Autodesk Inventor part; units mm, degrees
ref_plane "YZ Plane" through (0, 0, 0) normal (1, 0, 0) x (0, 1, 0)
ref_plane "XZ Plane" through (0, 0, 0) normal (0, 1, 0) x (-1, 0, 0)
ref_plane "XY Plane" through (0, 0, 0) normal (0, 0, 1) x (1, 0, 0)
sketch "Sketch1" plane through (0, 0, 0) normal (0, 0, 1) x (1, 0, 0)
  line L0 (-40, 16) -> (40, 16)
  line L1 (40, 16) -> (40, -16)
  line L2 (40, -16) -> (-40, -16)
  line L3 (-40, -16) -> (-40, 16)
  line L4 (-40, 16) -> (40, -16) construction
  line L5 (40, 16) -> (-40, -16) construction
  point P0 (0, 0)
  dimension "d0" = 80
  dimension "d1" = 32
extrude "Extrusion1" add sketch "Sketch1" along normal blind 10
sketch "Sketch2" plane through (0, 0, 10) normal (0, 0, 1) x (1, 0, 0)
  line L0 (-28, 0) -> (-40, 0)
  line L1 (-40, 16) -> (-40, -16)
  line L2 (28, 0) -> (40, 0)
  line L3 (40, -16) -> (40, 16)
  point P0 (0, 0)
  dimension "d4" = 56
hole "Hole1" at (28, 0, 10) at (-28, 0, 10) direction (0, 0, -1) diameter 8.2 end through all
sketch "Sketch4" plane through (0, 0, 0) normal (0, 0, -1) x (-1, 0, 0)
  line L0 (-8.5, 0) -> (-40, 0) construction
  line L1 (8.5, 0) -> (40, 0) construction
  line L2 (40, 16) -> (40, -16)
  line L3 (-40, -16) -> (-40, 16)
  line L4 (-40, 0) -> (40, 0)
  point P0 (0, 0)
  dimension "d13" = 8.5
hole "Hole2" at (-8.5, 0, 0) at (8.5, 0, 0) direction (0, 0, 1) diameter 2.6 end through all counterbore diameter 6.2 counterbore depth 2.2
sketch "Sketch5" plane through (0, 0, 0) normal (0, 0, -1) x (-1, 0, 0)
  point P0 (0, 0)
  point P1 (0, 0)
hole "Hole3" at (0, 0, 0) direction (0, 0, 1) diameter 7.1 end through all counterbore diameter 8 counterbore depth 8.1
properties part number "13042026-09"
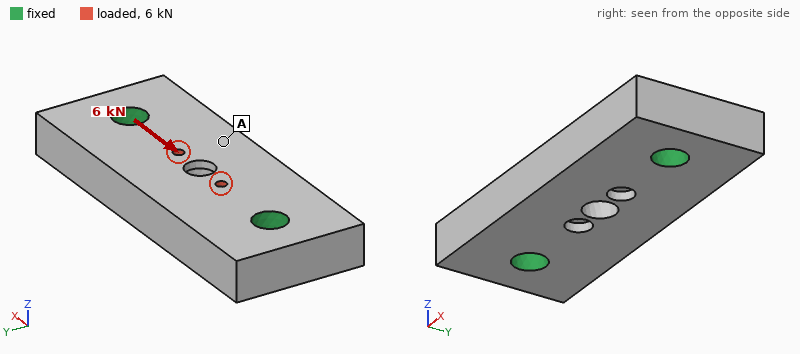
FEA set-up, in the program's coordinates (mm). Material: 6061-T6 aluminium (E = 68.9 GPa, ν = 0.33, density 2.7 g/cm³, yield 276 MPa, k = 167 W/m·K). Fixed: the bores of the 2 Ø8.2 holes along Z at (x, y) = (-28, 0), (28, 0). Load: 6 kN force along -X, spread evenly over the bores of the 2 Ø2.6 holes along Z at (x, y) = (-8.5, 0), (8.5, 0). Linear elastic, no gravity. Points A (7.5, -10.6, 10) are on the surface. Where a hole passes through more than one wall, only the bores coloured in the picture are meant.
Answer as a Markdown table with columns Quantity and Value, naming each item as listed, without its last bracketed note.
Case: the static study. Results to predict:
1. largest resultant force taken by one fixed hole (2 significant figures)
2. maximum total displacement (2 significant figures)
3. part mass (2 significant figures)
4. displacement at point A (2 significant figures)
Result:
| Quantity | Value |
|---|---|
| largest resultant force taken by one fixed hole | 3.0 kN |
| maximum total displacement | 7.2 µm |
| part mass | 64 g |
| displacement at point A | 2.8 µm |
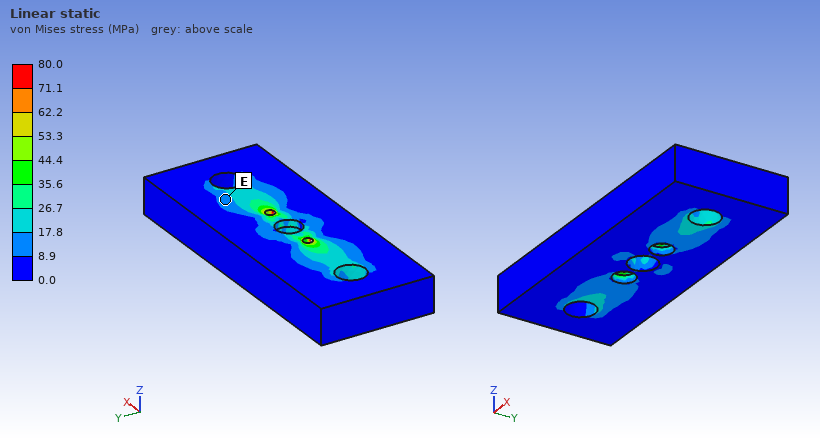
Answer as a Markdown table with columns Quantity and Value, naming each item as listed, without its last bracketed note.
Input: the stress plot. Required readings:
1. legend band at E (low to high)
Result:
| Quantity | Value |
|---|---|
| legend band at E | 8.9 to 17.8 MPa |
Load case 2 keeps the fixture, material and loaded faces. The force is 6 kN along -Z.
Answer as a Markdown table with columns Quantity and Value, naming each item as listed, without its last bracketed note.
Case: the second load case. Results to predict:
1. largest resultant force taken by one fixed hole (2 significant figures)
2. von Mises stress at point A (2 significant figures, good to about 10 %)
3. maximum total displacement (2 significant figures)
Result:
| Quantity | Value |
|---|---|
| largest resultant force taken by one fixed hole | 3.0 kN |
| von Mises stress at point A | 34 MPa |
| maximum total displacement | 36 µm |
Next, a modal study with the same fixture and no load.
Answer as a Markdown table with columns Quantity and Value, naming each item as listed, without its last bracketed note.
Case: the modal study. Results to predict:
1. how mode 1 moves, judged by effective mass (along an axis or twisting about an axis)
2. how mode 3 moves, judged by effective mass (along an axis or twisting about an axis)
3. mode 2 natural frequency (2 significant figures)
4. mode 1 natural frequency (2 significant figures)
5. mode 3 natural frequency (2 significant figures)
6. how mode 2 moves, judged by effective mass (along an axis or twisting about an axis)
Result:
| Quantity | Value |
|---|---|
| how mode 1 moves, judged by effective mass | along Z |
| how mode 3 moves, judged by effective mass | along Y |
| mode 2 natural frequency | 16 kHz |
| mode 1 natural frequency | 14 kHz |
| mode 3 natural frequency | 21 kHz |
| how mode 2 moves, judged by effective mass | twisting about X |
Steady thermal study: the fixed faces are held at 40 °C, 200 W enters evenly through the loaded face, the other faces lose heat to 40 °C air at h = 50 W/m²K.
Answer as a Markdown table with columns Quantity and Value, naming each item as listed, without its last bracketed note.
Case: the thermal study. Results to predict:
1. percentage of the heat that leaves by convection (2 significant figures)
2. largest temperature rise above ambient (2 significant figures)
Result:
| Quantity | Value |
|---|---|
| percentage of the heat that leaves by convection | 3.2 % |
| largest temperature rise above ambient | 57 K |
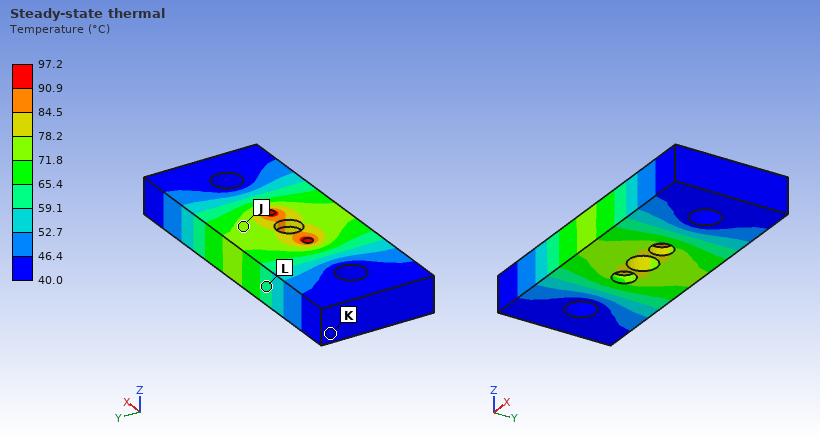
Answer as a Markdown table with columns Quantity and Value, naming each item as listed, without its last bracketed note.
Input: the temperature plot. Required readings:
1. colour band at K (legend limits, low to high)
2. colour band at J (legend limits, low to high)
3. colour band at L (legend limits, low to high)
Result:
| Quantity | Value |
|---|---|
| colour band at K | 40.0 to 46.4 °C |
| colour band at J | 71.8 to 78.2 °C |
| colour band at L | 59.1 to 65.4 °C |
